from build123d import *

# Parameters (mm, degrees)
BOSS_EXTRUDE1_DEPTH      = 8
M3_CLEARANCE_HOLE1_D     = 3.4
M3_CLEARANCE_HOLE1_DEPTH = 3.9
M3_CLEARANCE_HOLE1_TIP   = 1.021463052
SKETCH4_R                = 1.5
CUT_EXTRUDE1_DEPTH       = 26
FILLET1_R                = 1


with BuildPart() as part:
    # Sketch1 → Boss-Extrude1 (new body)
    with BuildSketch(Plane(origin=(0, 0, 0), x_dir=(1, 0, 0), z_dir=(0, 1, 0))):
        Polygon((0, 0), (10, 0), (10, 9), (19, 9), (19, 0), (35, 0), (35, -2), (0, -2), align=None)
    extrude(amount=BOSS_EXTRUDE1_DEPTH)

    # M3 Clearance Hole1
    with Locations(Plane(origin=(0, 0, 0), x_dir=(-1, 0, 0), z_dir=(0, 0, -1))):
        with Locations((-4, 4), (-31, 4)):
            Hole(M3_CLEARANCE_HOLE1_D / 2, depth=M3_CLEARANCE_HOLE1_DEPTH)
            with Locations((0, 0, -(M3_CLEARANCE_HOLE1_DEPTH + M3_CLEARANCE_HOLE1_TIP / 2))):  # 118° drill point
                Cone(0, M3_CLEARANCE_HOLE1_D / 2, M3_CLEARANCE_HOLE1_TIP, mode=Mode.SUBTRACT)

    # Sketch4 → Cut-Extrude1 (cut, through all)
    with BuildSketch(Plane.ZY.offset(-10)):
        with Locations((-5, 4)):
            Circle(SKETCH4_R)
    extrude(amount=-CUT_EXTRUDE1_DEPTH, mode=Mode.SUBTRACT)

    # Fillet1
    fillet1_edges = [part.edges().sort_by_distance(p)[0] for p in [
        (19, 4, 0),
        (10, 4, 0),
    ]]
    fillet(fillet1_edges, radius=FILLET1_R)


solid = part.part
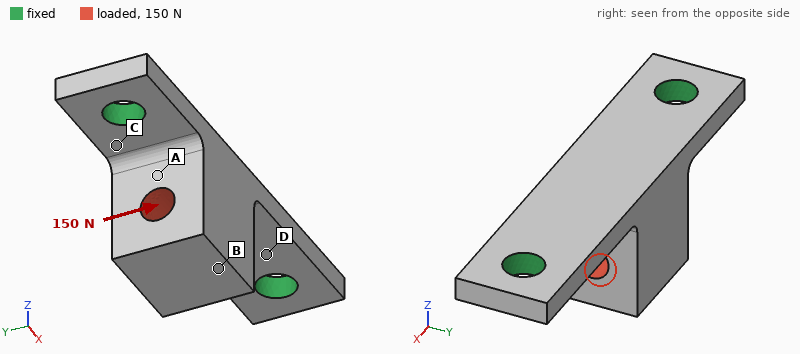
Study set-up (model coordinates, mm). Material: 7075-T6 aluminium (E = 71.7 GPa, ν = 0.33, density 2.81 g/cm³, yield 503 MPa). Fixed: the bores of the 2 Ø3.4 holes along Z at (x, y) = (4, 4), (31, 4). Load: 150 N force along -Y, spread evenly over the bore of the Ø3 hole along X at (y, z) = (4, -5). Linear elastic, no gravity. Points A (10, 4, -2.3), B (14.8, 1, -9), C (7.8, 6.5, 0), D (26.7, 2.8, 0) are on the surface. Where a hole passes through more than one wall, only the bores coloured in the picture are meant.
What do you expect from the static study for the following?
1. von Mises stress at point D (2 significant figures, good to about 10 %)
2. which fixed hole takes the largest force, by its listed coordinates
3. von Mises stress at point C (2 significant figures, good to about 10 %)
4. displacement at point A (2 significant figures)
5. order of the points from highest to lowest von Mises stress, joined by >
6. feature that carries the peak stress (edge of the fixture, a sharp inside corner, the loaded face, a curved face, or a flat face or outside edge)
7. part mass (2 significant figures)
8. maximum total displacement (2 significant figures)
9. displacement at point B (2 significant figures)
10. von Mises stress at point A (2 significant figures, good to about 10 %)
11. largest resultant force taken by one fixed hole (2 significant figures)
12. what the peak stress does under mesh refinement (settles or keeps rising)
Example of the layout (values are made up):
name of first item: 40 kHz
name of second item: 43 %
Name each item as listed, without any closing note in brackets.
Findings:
von Mises stress at point D: 47 MPa
which fixed hole takes the largest force, by its listed coordinates: (4, 4)
von Mises stress at point C: 79 MPa
displacement at point A: 19 µm
order of the points from highest to lowest von Mises stress, joined by >: C > D > A > B
feature that carries the peak stress: edge of the fixture
part mass: 3.1 g
maximum total displacement: 56 µm
displacement at point B: 54 µm
von Mises stress at point A: 19 MPa
largest resultant force taken by one fixed hole: 100 N
what the peak stress does under mesh refinement: keeps rising
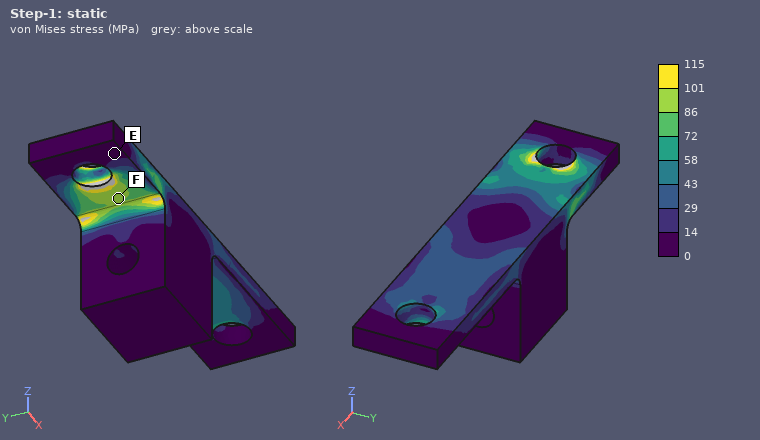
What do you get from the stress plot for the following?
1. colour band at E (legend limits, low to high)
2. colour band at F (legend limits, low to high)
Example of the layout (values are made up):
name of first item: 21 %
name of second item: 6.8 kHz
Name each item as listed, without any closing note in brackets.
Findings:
colour band at E: 0 to 14 MPa
colour band at F: 86 to 101 MPa
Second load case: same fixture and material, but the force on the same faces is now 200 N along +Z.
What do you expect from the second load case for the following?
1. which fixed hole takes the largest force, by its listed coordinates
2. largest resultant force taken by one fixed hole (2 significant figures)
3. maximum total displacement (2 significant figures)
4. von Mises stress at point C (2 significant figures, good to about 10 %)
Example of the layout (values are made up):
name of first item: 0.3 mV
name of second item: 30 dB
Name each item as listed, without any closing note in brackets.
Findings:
which fixed hole takes the largest force, by its listed coordinates: (4, 4)
largest resultant force taken by one fixed hole: 140 N
maximum total displacement: 24 µm
von Mises stress at point C: 11 MPa
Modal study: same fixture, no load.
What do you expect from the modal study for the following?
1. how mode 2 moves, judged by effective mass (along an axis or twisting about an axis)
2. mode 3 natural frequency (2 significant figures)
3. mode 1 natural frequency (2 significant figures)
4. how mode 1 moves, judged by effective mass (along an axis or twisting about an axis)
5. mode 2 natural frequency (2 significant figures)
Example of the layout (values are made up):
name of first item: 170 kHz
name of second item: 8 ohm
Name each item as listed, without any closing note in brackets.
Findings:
how mode 2 moves, judged by effective mass: along Z
mode 3 natural frequency: 22 kHz
mode 1 natural frequency: 7700 Hz
how mode 1 moves, judged by effective mass: along Y
mode 2 natural frequency: 10 kHz
